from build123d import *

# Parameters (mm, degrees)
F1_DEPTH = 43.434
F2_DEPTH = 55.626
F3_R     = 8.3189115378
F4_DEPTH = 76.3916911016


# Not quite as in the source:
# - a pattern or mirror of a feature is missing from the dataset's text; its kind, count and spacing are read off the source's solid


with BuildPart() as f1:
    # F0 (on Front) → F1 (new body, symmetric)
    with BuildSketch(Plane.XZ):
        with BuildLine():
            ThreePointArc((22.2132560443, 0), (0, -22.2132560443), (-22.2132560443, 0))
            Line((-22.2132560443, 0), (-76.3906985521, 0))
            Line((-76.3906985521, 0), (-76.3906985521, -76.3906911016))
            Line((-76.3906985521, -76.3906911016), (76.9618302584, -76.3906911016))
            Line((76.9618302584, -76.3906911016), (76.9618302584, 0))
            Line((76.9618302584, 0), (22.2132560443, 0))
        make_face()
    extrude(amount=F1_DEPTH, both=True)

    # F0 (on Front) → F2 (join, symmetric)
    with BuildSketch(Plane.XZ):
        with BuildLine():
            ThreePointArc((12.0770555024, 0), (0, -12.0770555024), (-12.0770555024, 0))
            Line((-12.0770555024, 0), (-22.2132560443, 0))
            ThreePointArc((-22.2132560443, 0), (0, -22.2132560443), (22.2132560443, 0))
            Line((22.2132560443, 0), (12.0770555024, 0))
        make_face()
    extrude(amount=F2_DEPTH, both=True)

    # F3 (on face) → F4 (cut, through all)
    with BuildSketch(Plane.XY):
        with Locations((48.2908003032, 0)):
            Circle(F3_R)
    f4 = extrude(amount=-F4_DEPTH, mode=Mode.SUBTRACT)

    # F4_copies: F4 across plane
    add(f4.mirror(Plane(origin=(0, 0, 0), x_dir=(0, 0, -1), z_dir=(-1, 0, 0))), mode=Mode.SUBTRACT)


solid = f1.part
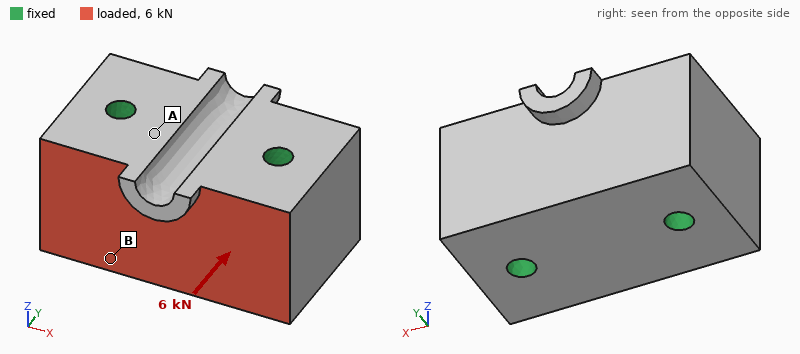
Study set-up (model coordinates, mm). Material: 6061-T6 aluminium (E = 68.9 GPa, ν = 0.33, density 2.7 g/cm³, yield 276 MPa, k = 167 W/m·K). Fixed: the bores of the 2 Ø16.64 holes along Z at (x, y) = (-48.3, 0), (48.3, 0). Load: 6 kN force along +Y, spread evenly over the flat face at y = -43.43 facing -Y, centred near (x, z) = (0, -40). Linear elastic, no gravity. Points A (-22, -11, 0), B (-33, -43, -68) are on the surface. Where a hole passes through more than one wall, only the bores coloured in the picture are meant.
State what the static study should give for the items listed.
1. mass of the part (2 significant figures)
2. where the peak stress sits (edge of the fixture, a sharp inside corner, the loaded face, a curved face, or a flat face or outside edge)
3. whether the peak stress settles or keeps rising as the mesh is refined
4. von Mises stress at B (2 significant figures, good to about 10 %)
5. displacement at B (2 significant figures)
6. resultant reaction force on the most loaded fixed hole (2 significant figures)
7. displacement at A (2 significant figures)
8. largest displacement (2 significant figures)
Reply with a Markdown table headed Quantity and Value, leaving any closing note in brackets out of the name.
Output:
| Quantity | Value |
|---|---|
| mass of the part | 2.6 kg |
| where the peak stress sits | edge of the fixture |
| whether the peak stress settles or keeps rising as the mesh is refined | keeps rising |
| von Mises stress at B | 0.57 MPa |
| displacement at B | 0.49 µm |
| resultant reaction force on the most loaded fixed hole | 3.0 kN |
| displacement at A | 0.25 µm |
| largest displacement | 0.67 µm |
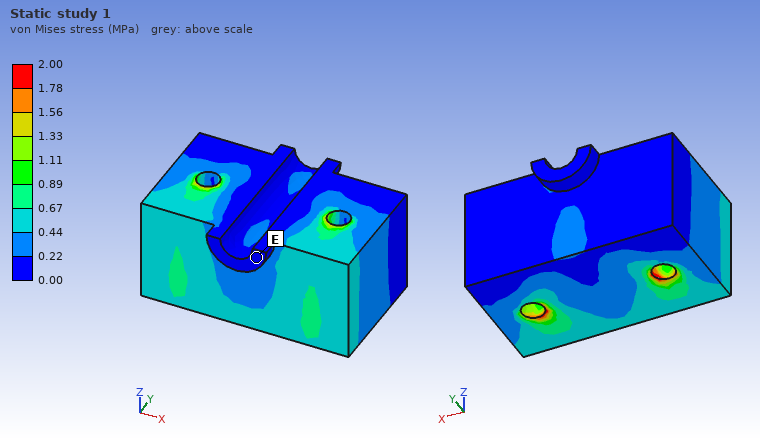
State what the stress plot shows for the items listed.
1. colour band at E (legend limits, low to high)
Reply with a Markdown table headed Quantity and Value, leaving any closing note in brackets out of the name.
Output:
| Quantity | Value |
|---|---|
| colour band at E | 0.00 to 0.22 MPa |
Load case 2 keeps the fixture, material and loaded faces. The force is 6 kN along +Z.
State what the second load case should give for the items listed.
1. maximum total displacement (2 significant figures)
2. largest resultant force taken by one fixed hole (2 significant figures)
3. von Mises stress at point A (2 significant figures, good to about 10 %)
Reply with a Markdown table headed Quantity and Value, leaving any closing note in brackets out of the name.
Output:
| Quantity | Value |
|---|---|
| maximum total displacement | 2.5 µm |
| largest resultant force taken by one fixed hole | 3.0 kN |
| von Mises stress at point A | 0.79 MPa |
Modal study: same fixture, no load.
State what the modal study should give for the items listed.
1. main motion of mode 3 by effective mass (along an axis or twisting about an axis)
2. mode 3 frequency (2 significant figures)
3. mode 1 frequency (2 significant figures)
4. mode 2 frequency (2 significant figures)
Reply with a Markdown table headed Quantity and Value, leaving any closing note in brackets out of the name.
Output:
| Quantity | Value |
|---|---|
| main motion of mode 3 by effective mass | along Y |
| mode 3 frequency | 12 kHz |
| mode 1 frequency | 11 kHz |
| mode 2 frequency | 11 kHz |
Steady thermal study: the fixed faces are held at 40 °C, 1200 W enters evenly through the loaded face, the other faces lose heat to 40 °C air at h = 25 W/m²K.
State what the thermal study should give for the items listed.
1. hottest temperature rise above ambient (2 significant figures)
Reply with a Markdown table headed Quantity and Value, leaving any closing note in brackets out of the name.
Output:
| Quantity | Value |
|---|---|
| hottest temperature rise above ambient | 33 K |
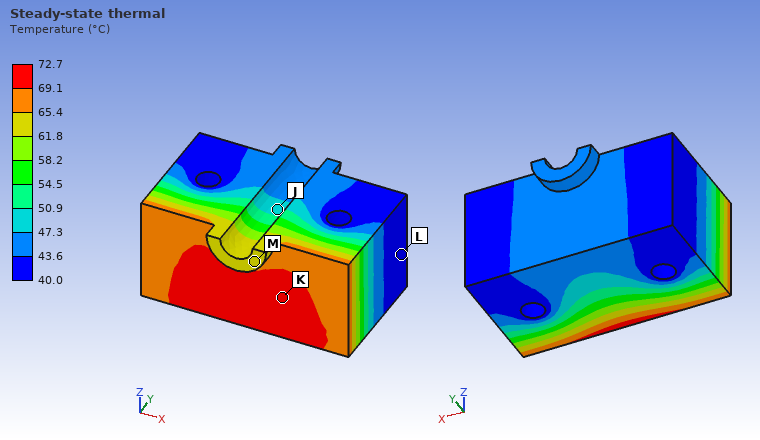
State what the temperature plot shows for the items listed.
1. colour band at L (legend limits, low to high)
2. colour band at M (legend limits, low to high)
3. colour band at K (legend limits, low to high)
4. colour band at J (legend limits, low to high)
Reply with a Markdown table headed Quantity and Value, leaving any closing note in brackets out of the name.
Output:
| Quantity | Value |
|---|---|
| colour band at L | 40.0 to 43.6 °C |
| colour band at M | 61.8 to 65.4 °C |
| colour band at K | 69.1 to 72.7 °C |
| colour band at J | 47.3 to 50.9 °C |
